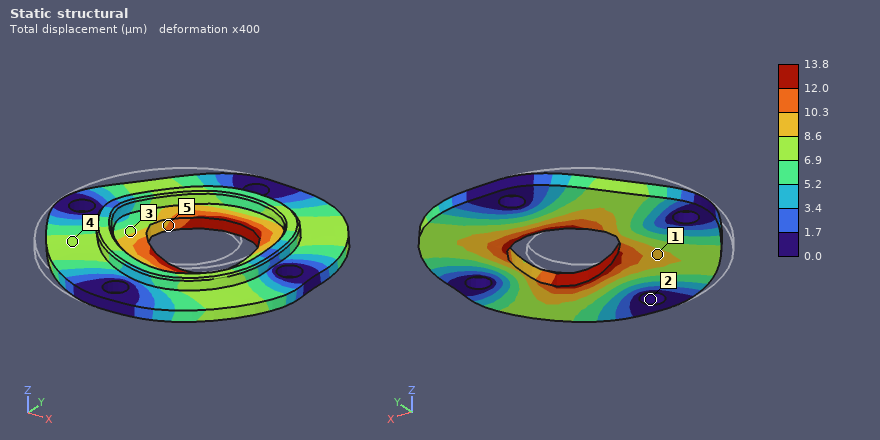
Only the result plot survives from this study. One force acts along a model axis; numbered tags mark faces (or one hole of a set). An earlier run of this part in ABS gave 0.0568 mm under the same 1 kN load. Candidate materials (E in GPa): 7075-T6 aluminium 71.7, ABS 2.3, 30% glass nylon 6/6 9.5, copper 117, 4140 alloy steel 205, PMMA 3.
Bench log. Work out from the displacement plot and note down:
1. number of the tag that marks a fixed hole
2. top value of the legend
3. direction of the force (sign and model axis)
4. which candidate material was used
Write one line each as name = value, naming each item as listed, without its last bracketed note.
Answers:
number of the tag that marks a fixed hole = 2
top value of the legend = 13.8 µm
direction of the force = +X
which candidate material was used = 30% glass nylon 6/6
